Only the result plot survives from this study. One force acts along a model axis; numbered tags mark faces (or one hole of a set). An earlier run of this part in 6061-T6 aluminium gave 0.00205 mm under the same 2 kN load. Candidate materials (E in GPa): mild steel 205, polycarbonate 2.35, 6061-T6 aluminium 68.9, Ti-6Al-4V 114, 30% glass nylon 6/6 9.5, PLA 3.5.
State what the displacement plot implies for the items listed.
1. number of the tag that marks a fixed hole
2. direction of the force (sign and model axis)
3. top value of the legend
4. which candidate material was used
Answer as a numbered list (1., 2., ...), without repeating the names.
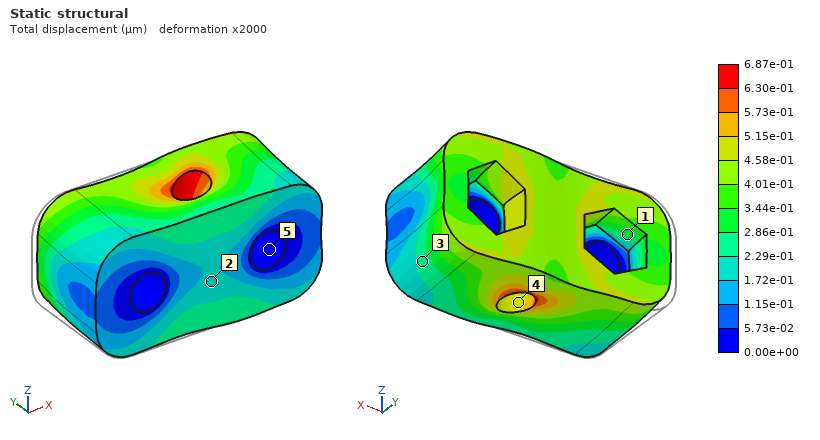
1. 5
2. +X
3. 6.87e-01 µm
4. mild steel
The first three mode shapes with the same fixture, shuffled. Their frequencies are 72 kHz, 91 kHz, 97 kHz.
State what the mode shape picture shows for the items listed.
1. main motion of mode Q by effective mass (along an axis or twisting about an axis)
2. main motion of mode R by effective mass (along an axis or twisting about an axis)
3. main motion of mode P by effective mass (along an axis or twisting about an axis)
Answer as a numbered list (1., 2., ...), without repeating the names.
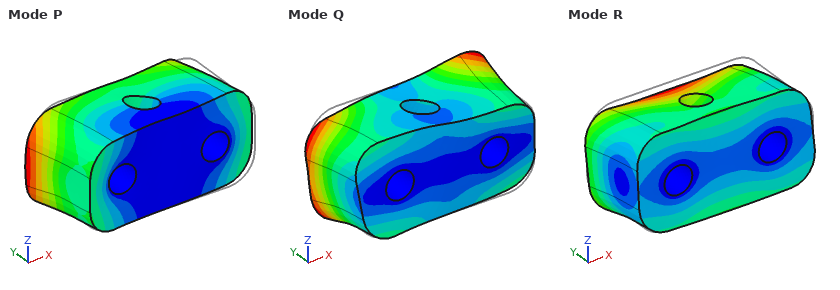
1. twisting about Y
2. along Z
3. along X
